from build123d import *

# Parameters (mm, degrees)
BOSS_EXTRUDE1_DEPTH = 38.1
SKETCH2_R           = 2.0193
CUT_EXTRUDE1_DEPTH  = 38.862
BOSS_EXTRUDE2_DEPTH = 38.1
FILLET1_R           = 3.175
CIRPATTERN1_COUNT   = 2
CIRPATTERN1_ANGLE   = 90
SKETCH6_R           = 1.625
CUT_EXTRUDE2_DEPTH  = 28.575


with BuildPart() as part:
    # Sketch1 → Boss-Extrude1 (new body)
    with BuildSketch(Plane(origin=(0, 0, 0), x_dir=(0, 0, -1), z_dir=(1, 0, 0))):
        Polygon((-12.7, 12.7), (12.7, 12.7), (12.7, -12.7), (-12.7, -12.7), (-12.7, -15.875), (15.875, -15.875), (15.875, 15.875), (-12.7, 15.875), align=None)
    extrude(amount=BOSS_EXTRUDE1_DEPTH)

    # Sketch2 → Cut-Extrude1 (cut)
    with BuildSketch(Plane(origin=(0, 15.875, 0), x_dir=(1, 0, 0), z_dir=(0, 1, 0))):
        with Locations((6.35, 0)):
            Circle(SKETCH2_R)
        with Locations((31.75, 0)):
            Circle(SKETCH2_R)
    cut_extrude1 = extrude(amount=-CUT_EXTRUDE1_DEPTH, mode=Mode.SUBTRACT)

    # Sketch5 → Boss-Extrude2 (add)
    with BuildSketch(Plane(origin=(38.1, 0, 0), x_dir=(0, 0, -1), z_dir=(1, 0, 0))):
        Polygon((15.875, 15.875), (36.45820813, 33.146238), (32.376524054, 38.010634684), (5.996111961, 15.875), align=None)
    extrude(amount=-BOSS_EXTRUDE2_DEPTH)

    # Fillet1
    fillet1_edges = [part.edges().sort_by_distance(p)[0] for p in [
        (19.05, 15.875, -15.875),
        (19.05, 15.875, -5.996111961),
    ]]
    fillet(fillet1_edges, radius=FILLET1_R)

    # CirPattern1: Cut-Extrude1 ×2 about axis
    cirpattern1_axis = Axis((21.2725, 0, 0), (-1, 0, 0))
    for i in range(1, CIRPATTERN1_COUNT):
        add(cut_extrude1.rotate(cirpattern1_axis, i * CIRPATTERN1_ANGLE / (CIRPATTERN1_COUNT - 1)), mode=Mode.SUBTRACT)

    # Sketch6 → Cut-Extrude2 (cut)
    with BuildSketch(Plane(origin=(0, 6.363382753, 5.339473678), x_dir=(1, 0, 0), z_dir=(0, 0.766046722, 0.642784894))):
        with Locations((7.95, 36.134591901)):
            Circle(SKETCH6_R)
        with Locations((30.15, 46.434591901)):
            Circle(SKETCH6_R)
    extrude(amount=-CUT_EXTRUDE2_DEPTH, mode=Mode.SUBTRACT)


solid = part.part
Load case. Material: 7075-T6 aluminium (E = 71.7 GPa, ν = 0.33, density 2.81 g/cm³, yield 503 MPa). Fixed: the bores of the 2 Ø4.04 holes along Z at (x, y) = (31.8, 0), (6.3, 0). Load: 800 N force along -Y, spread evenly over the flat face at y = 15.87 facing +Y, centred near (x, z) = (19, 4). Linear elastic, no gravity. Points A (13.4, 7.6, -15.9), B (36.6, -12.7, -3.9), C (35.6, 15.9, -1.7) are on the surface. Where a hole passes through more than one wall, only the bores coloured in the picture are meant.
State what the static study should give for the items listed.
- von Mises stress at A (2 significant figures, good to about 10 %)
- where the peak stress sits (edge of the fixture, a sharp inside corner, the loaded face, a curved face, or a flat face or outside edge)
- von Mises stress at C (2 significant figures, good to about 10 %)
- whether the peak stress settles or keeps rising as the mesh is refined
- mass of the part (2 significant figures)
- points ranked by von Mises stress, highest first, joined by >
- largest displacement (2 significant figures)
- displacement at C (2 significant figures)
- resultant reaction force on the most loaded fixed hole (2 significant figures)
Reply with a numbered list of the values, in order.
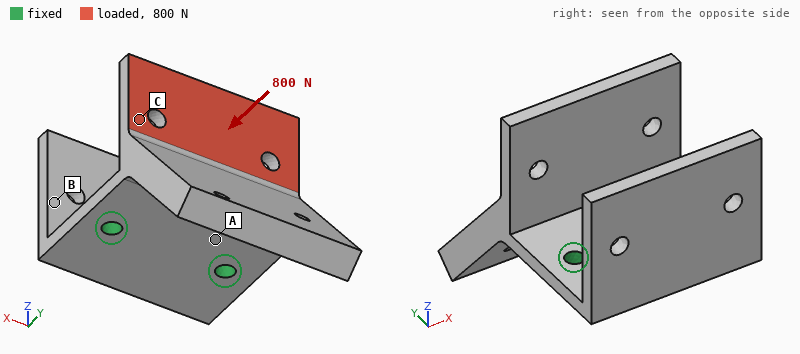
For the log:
1. 190 MPa
2. edge of the fixture
3. 93 MPa
4. keeps rising
5. 48 g
6. A > C > B
7. 0.95 mm
8. 0.43 mm
9. 400 N
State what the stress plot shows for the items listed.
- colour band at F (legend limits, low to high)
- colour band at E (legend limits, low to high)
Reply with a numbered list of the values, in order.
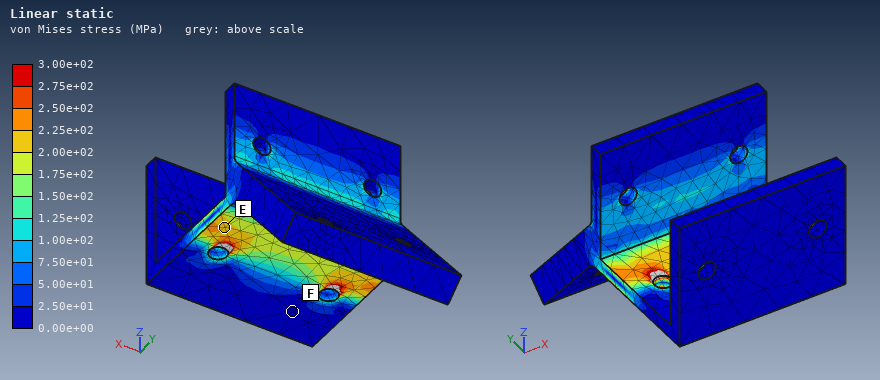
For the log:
1. 0.00e+00 to 2.50e+01 MPa
2. 2.00e+02 to 2.25e+02 MPa
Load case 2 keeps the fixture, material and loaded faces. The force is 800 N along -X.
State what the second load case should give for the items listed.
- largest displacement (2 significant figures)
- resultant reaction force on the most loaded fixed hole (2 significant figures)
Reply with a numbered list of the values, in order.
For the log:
1. 0.13 mm
2. 810 N
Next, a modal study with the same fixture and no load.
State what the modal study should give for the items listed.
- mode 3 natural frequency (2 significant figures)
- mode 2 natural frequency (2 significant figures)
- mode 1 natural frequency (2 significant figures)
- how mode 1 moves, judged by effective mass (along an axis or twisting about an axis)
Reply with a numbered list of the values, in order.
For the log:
1. 3200 Hz
2. 2000 Hz
3. 1000 Hz
4. along Z
